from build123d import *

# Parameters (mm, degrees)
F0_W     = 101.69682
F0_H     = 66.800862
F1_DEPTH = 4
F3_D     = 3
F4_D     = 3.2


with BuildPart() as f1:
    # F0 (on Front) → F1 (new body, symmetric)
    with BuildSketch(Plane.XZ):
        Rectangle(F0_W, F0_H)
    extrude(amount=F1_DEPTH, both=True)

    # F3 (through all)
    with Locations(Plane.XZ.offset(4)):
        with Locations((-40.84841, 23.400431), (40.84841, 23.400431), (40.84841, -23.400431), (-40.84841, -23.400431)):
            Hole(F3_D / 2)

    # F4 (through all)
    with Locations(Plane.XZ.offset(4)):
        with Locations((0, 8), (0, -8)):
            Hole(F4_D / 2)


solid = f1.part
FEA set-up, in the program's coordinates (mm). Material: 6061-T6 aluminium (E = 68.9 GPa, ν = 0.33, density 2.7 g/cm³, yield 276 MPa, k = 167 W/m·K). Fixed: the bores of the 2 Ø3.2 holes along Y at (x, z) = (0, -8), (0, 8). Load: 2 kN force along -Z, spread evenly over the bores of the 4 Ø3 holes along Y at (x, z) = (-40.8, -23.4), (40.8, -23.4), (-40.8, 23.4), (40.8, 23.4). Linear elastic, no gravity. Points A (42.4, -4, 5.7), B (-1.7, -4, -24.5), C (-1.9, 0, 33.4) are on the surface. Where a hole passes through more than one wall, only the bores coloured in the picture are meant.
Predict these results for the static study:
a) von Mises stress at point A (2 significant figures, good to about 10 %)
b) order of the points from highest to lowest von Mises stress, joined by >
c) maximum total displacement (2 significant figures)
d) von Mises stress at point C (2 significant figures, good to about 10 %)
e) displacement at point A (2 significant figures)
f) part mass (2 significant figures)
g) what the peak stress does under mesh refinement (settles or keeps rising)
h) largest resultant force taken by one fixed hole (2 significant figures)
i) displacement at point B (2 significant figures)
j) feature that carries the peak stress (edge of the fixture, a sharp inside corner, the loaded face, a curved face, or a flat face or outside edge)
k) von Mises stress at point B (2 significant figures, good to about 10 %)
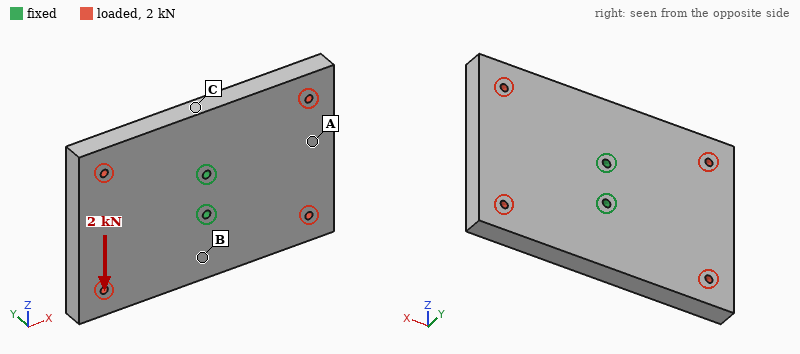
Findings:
2.2 MPa
C > B > A
7.1 µm
8.1 MPa
5.6 µm
150 g
keeps rising
1.0 kN
1.2 µm
edge of the fixture
5.0 MPa
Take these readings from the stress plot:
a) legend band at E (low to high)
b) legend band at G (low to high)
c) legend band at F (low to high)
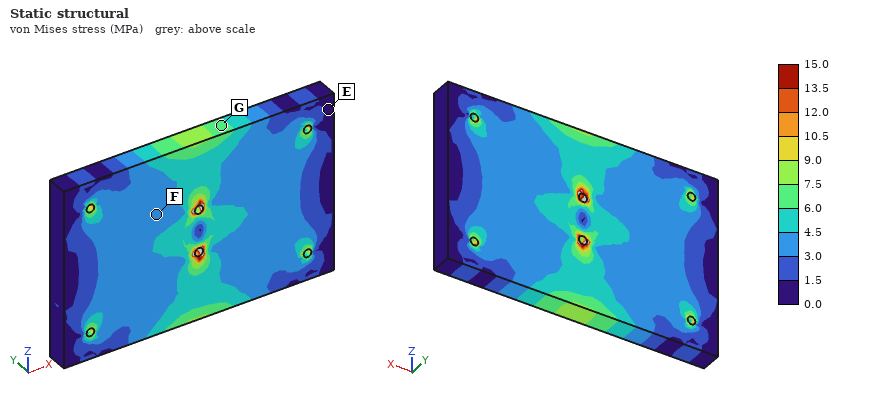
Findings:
0.0 to 1.5 MPa
6.0 to 7.5 MPa
3.0 to 4.5 MPa
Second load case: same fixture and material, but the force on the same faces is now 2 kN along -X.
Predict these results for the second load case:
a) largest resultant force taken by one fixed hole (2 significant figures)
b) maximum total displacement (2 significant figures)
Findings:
1.0 kN
2.9 µm
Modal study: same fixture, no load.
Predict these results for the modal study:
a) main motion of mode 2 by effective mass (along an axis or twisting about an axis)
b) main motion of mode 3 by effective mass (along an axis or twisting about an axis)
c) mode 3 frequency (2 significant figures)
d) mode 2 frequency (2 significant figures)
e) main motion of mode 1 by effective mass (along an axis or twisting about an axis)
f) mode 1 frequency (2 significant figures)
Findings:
along Y
twisting about X
3600 Hz
2600 Hz
twisting about Z
1800 Hz
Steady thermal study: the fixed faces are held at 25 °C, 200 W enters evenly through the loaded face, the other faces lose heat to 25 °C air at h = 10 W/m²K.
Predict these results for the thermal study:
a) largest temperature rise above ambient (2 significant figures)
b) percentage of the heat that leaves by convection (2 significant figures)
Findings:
75 K
3.8 %
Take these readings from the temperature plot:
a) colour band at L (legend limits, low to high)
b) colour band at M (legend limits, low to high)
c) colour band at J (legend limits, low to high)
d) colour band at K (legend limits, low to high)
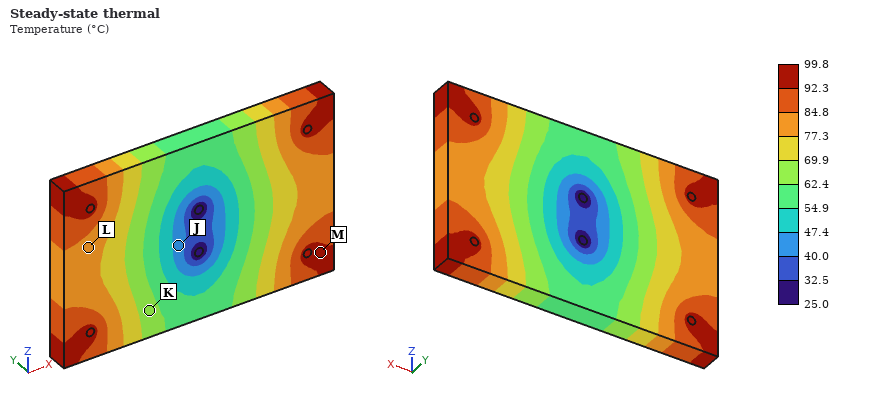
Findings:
77.3 to 84.8 °C
92.3 to 99.8 °C
40.0 to 47.4 °C
62.4 to 69.9 °C
